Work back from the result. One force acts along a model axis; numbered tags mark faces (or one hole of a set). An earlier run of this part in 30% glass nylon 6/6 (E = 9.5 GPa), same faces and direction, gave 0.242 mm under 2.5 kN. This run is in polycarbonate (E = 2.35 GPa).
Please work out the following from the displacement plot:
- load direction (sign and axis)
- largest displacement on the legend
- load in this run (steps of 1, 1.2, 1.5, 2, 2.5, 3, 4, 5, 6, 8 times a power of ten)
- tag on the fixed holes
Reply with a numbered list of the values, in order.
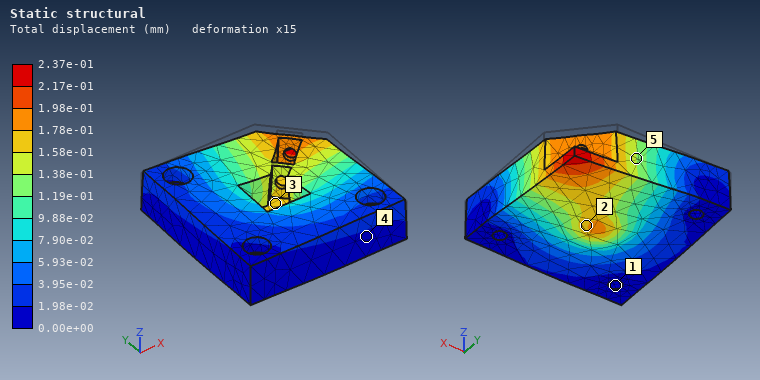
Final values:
1. -Z
2. 2.37e-01 mm
3. 600 N
4. 1
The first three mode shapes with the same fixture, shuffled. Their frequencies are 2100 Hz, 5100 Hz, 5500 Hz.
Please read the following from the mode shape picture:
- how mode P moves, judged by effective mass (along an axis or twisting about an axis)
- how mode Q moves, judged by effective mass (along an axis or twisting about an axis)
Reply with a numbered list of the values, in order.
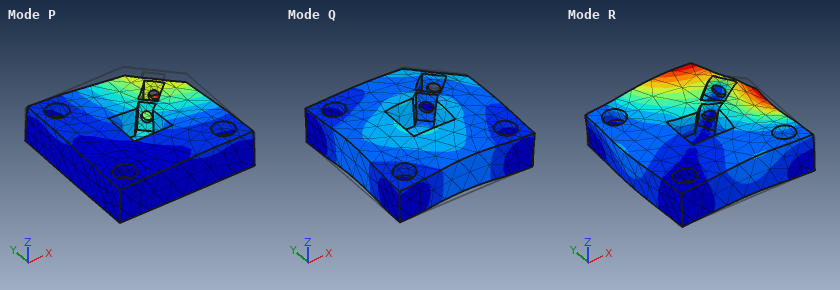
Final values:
1. along Z
2. along Z
